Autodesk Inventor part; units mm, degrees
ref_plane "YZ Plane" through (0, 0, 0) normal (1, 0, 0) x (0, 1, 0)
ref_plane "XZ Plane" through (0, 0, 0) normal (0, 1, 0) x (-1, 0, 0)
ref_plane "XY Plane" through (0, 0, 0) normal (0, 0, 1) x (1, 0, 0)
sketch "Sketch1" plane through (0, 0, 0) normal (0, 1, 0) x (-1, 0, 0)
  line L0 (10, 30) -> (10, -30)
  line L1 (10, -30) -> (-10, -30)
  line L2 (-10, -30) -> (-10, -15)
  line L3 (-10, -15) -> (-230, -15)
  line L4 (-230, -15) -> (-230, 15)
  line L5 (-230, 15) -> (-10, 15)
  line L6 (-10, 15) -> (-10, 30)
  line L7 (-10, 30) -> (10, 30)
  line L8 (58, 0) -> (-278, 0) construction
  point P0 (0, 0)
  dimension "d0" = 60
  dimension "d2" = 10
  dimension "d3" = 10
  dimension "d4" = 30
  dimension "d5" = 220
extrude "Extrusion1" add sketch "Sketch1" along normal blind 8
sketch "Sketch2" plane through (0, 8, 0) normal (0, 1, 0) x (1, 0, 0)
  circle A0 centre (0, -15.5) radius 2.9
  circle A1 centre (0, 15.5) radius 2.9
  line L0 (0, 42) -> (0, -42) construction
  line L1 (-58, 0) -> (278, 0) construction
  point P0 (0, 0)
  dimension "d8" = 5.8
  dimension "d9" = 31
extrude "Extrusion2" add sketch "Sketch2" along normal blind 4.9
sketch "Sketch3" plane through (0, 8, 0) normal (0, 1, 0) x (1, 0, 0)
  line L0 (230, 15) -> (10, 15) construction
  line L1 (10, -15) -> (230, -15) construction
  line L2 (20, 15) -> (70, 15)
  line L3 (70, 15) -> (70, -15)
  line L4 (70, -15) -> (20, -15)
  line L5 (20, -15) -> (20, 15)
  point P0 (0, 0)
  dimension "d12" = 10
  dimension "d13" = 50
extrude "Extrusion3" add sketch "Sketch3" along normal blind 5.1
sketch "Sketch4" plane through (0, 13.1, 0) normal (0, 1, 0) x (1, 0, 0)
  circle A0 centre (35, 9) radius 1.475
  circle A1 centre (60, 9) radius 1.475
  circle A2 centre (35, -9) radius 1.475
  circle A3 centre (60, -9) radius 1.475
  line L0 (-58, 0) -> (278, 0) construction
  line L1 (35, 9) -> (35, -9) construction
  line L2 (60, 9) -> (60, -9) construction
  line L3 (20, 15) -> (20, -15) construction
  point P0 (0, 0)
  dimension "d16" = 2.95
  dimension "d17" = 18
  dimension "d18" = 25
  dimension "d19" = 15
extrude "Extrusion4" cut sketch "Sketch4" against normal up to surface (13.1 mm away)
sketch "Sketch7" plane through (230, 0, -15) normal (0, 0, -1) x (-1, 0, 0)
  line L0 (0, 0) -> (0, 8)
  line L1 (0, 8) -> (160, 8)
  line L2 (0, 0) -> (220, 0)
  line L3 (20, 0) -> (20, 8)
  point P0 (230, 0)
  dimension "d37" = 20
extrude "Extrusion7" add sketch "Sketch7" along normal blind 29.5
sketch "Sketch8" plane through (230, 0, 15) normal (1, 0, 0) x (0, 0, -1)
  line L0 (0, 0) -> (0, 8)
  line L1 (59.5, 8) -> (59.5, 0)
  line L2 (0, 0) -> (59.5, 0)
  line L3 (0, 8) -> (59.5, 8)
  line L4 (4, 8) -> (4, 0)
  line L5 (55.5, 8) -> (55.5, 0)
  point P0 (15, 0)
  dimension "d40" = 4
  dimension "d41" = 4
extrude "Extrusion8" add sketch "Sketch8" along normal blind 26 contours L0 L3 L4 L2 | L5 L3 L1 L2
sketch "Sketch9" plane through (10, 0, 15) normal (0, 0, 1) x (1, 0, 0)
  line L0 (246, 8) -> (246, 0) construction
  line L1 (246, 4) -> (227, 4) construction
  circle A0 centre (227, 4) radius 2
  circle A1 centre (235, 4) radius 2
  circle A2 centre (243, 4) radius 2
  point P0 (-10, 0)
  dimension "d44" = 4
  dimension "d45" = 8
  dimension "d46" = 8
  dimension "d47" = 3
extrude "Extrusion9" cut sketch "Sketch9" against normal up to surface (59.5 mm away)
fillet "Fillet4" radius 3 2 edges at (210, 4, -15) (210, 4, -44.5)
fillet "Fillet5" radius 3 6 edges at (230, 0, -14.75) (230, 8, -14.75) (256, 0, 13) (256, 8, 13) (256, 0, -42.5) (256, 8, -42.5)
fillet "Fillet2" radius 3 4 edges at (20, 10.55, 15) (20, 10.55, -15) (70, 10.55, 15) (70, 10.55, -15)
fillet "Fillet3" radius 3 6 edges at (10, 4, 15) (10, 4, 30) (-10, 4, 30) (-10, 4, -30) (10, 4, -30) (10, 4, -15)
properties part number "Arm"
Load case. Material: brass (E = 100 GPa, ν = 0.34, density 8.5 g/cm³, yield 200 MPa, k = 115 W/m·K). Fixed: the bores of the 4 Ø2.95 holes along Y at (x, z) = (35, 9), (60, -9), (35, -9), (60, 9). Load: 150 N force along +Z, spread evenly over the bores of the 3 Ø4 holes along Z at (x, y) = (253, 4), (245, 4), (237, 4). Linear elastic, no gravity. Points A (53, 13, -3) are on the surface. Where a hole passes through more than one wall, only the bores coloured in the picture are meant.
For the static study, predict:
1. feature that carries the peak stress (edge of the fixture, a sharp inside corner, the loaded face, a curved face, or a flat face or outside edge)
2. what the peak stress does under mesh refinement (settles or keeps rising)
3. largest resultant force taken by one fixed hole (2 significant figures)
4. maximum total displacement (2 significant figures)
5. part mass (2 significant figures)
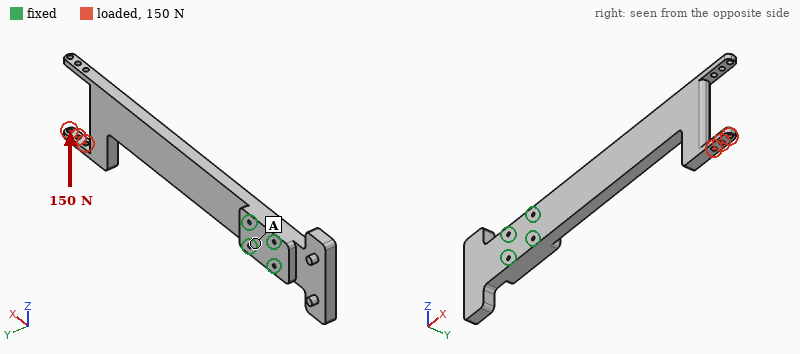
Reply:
a sharp inside corner
keeps rising
1.2 kN
0.38 mm
640 g
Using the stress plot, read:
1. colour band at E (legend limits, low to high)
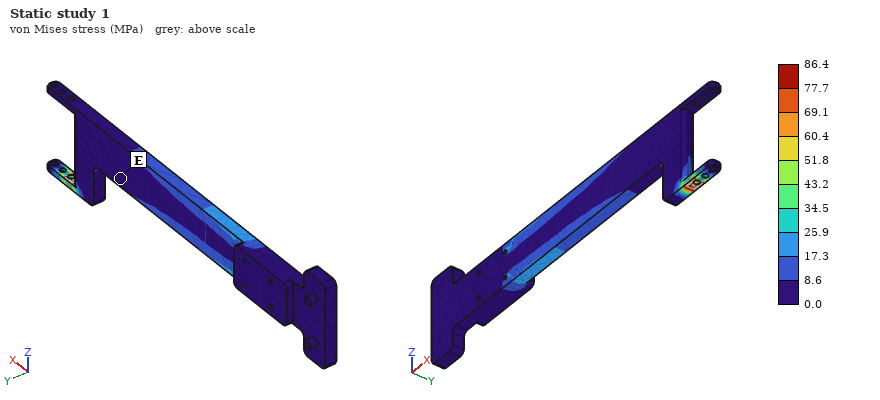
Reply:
0.0 to 8.6 MPa
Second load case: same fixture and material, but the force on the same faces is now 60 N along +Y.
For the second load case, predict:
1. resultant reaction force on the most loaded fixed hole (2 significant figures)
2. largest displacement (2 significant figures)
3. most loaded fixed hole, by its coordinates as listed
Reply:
190 N
1.1 mm
(60, -9)
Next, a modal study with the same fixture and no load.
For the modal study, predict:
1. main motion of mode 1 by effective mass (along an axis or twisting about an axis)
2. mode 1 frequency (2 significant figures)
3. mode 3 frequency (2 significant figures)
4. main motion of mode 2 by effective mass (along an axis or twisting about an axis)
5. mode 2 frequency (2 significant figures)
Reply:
along Y
130 Hz
710 Hz
along Z
450 Hz
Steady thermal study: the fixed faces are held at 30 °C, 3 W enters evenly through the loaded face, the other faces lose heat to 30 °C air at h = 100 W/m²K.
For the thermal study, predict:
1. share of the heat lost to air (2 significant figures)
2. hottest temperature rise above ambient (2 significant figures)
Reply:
95 %
20 K
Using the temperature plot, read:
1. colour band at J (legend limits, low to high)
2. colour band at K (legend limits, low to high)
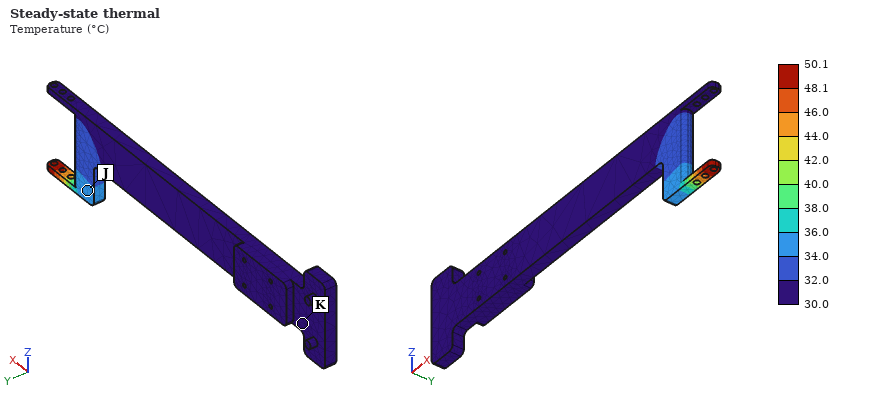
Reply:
34.0 to 36.0 °C
30.0 to 32.0 °C
